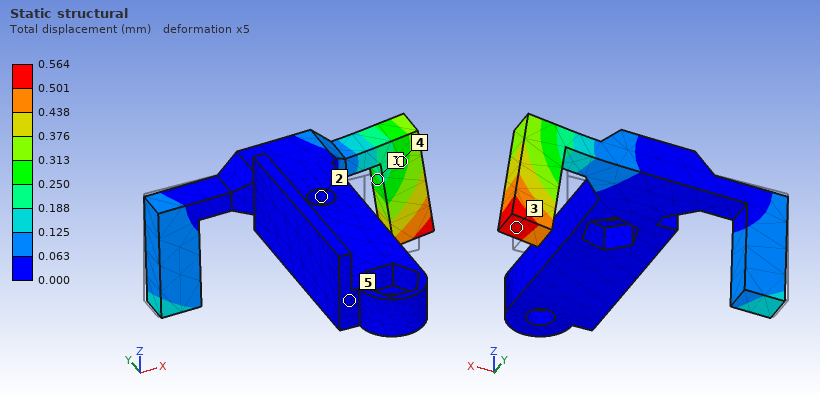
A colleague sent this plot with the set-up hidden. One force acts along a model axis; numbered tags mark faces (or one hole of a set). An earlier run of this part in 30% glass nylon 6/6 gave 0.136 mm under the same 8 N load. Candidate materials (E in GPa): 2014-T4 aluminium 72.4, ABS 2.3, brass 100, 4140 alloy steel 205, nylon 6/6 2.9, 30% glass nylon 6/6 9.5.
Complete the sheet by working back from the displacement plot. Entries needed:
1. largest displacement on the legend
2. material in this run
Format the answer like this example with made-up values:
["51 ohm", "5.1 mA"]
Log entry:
["0.564 mm", "ABS"]
